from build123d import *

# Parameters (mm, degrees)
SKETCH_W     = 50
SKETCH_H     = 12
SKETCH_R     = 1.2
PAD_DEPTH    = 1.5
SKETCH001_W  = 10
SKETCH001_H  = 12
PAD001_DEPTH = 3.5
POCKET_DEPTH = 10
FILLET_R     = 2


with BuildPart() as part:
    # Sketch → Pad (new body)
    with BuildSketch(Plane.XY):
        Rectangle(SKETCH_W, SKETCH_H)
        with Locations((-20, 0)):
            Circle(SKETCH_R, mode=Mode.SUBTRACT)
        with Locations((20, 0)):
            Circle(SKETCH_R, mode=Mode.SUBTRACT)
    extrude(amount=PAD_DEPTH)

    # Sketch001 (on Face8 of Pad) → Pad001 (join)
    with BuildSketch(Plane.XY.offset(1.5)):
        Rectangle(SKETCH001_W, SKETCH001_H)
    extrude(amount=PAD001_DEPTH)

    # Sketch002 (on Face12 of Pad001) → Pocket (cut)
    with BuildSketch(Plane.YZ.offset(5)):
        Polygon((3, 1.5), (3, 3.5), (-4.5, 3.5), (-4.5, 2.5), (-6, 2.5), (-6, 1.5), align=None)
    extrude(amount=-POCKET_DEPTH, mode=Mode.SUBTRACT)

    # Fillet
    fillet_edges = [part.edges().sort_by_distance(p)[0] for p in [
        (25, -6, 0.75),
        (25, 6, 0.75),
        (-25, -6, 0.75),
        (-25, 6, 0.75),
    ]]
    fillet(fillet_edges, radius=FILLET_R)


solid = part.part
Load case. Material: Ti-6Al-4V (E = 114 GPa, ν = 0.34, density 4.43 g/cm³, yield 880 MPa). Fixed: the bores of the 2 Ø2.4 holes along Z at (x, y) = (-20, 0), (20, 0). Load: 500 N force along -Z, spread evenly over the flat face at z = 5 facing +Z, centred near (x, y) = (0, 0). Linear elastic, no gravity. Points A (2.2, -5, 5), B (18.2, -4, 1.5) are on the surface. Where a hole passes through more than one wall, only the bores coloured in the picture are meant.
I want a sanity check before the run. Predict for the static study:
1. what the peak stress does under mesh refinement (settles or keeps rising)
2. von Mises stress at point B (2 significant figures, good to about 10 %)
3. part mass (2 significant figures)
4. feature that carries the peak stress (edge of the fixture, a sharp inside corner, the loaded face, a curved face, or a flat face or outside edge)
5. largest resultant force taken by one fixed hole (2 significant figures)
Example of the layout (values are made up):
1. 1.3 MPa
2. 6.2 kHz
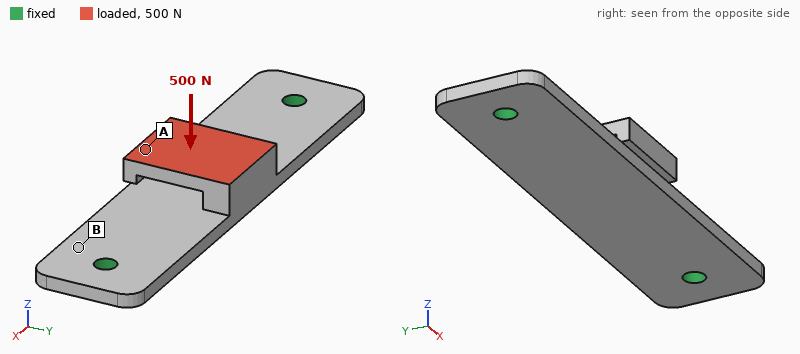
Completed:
1. keeps rising
2. 260 MPa
3. 5.0 g
4. edge of the fixture
5. 260 N
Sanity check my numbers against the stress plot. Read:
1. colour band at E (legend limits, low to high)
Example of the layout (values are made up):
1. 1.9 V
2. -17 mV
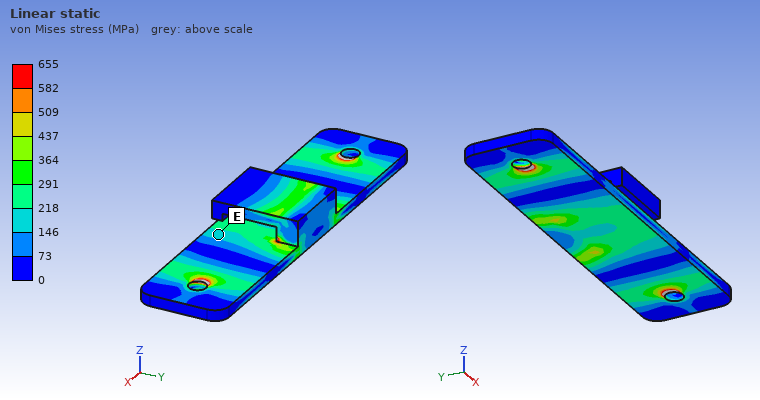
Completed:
1. 146 to 218 MPa
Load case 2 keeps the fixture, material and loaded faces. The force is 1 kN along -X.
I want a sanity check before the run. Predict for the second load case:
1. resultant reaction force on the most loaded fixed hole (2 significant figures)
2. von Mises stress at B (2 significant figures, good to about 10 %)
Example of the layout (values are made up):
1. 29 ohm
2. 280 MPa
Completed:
1. 520 N
2. 66 MPa
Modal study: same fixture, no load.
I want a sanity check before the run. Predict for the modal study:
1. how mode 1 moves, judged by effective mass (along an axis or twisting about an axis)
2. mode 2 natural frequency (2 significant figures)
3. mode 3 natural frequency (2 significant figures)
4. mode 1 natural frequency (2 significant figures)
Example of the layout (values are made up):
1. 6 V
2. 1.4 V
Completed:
1. along Z
2. 5900 Hz
3. 11 kHz
4. 4200 Hz
